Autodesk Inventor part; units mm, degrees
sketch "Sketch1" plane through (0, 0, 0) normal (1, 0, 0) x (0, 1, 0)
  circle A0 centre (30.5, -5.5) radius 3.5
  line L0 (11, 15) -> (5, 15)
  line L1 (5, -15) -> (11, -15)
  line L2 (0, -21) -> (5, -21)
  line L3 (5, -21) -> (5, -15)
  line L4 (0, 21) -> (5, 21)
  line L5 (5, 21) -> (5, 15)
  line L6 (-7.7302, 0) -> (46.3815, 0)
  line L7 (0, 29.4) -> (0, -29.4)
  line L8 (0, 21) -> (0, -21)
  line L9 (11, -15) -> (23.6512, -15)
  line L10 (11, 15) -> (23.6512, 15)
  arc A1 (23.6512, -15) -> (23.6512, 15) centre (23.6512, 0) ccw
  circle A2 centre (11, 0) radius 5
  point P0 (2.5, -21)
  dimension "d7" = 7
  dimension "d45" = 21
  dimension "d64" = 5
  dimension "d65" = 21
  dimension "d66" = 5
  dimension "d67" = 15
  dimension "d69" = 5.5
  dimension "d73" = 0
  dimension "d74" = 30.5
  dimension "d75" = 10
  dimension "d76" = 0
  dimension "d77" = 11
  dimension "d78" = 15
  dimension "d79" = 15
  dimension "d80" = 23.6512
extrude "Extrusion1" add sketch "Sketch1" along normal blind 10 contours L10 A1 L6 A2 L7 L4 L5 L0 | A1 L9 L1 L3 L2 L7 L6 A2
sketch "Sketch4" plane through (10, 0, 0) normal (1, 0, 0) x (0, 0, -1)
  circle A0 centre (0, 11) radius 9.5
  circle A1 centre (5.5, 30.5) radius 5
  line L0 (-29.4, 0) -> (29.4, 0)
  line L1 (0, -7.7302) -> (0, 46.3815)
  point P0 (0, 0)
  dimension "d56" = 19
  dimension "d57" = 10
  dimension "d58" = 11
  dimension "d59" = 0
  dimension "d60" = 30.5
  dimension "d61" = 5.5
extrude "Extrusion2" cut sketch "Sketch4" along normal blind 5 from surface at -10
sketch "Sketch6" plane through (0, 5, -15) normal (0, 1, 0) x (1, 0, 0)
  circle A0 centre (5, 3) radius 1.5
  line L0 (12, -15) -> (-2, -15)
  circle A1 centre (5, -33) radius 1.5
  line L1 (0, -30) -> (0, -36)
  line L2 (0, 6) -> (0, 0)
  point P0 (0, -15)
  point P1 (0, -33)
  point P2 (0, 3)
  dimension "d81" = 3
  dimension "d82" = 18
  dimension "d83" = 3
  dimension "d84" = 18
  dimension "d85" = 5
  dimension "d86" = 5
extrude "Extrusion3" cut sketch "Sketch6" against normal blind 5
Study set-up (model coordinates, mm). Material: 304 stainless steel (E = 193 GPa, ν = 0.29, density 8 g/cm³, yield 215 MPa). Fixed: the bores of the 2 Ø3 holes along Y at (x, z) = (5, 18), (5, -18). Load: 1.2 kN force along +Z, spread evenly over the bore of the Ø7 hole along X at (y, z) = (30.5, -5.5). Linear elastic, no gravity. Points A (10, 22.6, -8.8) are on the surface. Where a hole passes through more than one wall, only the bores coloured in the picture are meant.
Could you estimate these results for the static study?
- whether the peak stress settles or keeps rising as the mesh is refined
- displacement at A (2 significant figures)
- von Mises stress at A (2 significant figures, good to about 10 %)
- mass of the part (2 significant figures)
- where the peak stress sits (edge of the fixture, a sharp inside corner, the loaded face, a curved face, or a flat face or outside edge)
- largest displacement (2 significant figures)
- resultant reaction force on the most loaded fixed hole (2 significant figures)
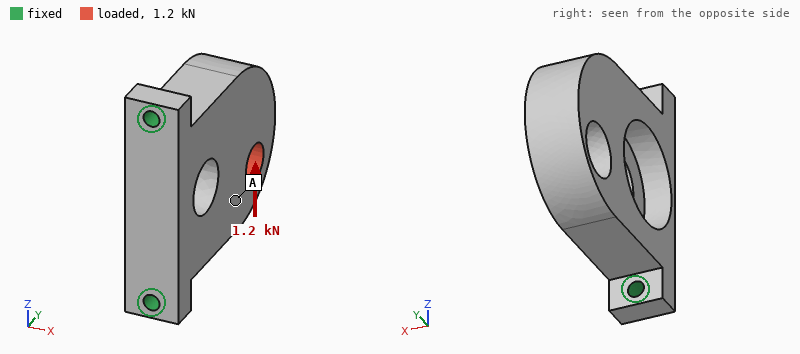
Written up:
keeps rising
6.6 µm
9.6 MPa
70 g
edge of the fixture
11 µm
1.2 kN
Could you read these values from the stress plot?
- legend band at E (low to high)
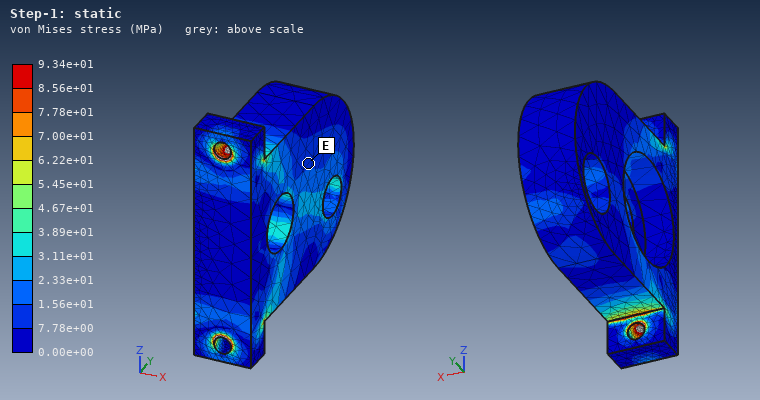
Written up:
7.78e+00 to 1.56e+01 MPa
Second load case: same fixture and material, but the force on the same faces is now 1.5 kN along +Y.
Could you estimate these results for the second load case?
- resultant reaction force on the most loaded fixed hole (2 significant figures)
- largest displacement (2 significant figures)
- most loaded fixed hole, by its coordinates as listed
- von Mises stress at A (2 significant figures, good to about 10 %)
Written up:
1.0 kN
21 µm
(5, -18)
21 MPa
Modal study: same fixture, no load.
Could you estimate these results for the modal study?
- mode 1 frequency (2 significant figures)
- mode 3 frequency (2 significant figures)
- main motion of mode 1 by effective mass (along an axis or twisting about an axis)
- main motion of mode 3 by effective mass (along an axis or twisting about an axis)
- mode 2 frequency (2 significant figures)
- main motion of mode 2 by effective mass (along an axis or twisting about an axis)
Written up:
2800 Hz
12 kHz
along X
along Z
9700 Hz
along Z
